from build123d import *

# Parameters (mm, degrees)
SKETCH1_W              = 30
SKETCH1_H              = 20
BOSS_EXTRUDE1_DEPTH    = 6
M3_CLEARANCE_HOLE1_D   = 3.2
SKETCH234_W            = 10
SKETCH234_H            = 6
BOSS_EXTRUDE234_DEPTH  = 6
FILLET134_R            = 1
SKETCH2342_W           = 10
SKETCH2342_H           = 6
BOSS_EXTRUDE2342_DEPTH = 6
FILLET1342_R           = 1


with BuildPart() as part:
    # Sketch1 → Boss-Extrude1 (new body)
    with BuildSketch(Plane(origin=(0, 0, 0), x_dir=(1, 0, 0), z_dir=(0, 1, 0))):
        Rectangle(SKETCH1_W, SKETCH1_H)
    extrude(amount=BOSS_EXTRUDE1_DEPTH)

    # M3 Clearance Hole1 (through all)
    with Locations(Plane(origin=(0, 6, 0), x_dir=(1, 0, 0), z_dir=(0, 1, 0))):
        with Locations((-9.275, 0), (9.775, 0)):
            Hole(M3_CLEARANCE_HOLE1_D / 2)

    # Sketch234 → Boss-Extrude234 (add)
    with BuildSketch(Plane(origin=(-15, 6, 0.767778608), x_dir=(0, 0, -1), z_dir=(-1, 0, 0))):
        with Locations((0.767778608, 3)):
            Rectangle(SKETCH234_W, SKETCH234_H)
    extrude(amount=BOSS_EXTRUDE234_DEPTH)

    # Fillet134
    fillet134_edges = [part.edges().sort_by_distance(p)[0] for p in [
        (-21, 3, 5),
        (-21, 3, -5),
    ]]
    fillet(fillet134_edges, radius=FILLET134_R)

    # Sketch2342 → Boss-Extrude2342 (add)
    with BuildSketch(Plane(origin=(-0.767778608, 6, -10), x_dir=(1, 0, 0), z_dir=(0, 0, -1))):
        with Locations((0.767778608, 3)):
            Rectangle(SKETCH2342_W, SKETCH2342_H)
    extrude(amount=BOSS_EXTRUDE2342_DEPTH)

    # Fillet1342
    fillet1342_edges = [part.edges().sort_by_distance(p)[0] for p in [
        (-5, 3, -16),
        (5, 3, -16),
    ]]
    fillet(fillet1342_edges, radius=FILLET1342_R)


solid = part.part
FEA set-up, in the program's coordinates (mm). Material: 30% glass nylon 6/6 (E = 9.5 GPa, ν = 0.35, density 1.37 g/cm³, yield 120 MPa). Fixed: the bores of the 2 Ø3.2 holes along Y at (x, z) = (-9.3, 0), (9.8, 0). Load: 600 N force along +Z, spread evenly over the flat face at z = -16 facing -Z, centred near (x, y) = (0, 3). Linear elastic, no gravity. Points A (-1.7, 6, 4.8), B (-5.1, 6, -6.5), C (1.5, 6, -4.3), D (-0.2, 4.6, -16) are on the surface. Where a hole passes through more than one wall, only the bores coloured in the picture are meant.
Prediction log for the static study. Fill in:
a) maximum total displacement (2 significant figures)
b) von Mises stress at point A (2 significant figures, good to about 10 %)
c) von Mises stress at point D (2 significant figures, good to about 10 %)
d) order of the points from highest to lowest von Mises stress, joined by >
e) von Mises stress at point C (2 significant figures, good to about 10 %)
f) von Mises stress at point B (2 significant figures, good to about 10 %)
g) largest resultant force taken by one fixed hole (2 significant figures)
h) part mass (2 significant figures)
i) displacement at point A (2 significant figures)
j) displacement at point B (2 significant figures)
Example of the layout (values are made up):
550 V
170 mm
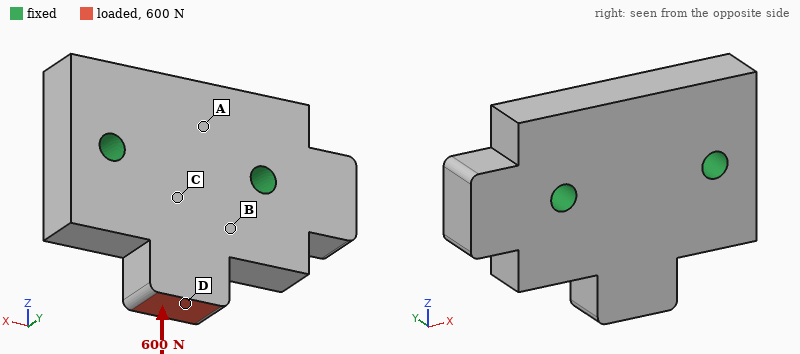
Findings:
18 µm
2.2 MPa
11 MPa
D > B > C > A
5.1 MPa
8.1 MPa
320 N
5.8 g
4.1 µm
5.9 µm
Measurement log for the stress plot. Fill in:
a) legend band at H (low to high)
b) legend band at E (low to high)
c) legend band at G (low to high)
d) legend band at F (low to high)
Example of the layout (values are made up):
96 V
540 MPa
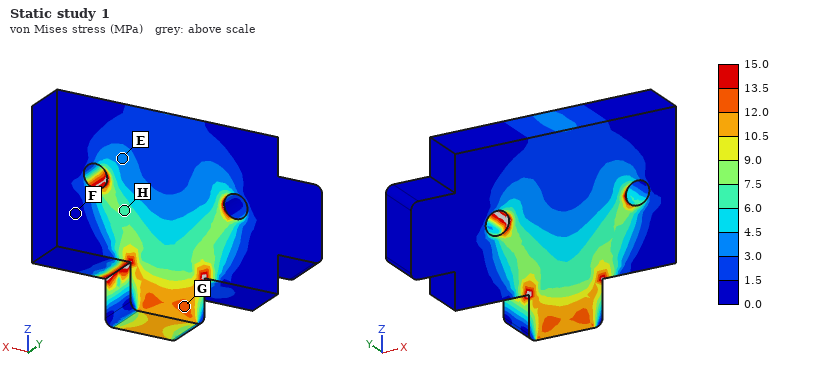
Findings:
6.0 to 7.5 MPa
3.0 to 4.5 MPa
12.0 to 13.5 MPa
0.0 to 1.5 MPa
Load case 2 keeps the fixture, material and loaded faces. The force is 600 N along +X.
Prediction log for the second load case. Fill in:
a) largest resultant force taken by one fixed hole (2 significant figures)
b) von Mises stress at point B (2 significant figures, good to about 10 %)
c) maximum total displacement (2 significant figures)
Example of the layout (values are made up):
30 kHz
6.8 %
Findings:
560 N
18 MPa
67 µm
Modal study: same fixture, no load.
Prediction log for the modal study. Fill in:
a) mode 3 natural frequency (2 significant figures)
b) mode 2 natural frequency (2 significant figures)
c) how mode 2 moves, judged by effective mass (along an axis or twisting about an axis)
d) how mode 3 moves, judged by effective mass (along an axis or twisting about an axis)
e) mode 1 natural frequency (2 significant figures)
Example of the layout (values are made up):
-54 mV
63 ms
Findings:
19 kHz
17 kHz
twisting about Z
along Y
11 kHz
